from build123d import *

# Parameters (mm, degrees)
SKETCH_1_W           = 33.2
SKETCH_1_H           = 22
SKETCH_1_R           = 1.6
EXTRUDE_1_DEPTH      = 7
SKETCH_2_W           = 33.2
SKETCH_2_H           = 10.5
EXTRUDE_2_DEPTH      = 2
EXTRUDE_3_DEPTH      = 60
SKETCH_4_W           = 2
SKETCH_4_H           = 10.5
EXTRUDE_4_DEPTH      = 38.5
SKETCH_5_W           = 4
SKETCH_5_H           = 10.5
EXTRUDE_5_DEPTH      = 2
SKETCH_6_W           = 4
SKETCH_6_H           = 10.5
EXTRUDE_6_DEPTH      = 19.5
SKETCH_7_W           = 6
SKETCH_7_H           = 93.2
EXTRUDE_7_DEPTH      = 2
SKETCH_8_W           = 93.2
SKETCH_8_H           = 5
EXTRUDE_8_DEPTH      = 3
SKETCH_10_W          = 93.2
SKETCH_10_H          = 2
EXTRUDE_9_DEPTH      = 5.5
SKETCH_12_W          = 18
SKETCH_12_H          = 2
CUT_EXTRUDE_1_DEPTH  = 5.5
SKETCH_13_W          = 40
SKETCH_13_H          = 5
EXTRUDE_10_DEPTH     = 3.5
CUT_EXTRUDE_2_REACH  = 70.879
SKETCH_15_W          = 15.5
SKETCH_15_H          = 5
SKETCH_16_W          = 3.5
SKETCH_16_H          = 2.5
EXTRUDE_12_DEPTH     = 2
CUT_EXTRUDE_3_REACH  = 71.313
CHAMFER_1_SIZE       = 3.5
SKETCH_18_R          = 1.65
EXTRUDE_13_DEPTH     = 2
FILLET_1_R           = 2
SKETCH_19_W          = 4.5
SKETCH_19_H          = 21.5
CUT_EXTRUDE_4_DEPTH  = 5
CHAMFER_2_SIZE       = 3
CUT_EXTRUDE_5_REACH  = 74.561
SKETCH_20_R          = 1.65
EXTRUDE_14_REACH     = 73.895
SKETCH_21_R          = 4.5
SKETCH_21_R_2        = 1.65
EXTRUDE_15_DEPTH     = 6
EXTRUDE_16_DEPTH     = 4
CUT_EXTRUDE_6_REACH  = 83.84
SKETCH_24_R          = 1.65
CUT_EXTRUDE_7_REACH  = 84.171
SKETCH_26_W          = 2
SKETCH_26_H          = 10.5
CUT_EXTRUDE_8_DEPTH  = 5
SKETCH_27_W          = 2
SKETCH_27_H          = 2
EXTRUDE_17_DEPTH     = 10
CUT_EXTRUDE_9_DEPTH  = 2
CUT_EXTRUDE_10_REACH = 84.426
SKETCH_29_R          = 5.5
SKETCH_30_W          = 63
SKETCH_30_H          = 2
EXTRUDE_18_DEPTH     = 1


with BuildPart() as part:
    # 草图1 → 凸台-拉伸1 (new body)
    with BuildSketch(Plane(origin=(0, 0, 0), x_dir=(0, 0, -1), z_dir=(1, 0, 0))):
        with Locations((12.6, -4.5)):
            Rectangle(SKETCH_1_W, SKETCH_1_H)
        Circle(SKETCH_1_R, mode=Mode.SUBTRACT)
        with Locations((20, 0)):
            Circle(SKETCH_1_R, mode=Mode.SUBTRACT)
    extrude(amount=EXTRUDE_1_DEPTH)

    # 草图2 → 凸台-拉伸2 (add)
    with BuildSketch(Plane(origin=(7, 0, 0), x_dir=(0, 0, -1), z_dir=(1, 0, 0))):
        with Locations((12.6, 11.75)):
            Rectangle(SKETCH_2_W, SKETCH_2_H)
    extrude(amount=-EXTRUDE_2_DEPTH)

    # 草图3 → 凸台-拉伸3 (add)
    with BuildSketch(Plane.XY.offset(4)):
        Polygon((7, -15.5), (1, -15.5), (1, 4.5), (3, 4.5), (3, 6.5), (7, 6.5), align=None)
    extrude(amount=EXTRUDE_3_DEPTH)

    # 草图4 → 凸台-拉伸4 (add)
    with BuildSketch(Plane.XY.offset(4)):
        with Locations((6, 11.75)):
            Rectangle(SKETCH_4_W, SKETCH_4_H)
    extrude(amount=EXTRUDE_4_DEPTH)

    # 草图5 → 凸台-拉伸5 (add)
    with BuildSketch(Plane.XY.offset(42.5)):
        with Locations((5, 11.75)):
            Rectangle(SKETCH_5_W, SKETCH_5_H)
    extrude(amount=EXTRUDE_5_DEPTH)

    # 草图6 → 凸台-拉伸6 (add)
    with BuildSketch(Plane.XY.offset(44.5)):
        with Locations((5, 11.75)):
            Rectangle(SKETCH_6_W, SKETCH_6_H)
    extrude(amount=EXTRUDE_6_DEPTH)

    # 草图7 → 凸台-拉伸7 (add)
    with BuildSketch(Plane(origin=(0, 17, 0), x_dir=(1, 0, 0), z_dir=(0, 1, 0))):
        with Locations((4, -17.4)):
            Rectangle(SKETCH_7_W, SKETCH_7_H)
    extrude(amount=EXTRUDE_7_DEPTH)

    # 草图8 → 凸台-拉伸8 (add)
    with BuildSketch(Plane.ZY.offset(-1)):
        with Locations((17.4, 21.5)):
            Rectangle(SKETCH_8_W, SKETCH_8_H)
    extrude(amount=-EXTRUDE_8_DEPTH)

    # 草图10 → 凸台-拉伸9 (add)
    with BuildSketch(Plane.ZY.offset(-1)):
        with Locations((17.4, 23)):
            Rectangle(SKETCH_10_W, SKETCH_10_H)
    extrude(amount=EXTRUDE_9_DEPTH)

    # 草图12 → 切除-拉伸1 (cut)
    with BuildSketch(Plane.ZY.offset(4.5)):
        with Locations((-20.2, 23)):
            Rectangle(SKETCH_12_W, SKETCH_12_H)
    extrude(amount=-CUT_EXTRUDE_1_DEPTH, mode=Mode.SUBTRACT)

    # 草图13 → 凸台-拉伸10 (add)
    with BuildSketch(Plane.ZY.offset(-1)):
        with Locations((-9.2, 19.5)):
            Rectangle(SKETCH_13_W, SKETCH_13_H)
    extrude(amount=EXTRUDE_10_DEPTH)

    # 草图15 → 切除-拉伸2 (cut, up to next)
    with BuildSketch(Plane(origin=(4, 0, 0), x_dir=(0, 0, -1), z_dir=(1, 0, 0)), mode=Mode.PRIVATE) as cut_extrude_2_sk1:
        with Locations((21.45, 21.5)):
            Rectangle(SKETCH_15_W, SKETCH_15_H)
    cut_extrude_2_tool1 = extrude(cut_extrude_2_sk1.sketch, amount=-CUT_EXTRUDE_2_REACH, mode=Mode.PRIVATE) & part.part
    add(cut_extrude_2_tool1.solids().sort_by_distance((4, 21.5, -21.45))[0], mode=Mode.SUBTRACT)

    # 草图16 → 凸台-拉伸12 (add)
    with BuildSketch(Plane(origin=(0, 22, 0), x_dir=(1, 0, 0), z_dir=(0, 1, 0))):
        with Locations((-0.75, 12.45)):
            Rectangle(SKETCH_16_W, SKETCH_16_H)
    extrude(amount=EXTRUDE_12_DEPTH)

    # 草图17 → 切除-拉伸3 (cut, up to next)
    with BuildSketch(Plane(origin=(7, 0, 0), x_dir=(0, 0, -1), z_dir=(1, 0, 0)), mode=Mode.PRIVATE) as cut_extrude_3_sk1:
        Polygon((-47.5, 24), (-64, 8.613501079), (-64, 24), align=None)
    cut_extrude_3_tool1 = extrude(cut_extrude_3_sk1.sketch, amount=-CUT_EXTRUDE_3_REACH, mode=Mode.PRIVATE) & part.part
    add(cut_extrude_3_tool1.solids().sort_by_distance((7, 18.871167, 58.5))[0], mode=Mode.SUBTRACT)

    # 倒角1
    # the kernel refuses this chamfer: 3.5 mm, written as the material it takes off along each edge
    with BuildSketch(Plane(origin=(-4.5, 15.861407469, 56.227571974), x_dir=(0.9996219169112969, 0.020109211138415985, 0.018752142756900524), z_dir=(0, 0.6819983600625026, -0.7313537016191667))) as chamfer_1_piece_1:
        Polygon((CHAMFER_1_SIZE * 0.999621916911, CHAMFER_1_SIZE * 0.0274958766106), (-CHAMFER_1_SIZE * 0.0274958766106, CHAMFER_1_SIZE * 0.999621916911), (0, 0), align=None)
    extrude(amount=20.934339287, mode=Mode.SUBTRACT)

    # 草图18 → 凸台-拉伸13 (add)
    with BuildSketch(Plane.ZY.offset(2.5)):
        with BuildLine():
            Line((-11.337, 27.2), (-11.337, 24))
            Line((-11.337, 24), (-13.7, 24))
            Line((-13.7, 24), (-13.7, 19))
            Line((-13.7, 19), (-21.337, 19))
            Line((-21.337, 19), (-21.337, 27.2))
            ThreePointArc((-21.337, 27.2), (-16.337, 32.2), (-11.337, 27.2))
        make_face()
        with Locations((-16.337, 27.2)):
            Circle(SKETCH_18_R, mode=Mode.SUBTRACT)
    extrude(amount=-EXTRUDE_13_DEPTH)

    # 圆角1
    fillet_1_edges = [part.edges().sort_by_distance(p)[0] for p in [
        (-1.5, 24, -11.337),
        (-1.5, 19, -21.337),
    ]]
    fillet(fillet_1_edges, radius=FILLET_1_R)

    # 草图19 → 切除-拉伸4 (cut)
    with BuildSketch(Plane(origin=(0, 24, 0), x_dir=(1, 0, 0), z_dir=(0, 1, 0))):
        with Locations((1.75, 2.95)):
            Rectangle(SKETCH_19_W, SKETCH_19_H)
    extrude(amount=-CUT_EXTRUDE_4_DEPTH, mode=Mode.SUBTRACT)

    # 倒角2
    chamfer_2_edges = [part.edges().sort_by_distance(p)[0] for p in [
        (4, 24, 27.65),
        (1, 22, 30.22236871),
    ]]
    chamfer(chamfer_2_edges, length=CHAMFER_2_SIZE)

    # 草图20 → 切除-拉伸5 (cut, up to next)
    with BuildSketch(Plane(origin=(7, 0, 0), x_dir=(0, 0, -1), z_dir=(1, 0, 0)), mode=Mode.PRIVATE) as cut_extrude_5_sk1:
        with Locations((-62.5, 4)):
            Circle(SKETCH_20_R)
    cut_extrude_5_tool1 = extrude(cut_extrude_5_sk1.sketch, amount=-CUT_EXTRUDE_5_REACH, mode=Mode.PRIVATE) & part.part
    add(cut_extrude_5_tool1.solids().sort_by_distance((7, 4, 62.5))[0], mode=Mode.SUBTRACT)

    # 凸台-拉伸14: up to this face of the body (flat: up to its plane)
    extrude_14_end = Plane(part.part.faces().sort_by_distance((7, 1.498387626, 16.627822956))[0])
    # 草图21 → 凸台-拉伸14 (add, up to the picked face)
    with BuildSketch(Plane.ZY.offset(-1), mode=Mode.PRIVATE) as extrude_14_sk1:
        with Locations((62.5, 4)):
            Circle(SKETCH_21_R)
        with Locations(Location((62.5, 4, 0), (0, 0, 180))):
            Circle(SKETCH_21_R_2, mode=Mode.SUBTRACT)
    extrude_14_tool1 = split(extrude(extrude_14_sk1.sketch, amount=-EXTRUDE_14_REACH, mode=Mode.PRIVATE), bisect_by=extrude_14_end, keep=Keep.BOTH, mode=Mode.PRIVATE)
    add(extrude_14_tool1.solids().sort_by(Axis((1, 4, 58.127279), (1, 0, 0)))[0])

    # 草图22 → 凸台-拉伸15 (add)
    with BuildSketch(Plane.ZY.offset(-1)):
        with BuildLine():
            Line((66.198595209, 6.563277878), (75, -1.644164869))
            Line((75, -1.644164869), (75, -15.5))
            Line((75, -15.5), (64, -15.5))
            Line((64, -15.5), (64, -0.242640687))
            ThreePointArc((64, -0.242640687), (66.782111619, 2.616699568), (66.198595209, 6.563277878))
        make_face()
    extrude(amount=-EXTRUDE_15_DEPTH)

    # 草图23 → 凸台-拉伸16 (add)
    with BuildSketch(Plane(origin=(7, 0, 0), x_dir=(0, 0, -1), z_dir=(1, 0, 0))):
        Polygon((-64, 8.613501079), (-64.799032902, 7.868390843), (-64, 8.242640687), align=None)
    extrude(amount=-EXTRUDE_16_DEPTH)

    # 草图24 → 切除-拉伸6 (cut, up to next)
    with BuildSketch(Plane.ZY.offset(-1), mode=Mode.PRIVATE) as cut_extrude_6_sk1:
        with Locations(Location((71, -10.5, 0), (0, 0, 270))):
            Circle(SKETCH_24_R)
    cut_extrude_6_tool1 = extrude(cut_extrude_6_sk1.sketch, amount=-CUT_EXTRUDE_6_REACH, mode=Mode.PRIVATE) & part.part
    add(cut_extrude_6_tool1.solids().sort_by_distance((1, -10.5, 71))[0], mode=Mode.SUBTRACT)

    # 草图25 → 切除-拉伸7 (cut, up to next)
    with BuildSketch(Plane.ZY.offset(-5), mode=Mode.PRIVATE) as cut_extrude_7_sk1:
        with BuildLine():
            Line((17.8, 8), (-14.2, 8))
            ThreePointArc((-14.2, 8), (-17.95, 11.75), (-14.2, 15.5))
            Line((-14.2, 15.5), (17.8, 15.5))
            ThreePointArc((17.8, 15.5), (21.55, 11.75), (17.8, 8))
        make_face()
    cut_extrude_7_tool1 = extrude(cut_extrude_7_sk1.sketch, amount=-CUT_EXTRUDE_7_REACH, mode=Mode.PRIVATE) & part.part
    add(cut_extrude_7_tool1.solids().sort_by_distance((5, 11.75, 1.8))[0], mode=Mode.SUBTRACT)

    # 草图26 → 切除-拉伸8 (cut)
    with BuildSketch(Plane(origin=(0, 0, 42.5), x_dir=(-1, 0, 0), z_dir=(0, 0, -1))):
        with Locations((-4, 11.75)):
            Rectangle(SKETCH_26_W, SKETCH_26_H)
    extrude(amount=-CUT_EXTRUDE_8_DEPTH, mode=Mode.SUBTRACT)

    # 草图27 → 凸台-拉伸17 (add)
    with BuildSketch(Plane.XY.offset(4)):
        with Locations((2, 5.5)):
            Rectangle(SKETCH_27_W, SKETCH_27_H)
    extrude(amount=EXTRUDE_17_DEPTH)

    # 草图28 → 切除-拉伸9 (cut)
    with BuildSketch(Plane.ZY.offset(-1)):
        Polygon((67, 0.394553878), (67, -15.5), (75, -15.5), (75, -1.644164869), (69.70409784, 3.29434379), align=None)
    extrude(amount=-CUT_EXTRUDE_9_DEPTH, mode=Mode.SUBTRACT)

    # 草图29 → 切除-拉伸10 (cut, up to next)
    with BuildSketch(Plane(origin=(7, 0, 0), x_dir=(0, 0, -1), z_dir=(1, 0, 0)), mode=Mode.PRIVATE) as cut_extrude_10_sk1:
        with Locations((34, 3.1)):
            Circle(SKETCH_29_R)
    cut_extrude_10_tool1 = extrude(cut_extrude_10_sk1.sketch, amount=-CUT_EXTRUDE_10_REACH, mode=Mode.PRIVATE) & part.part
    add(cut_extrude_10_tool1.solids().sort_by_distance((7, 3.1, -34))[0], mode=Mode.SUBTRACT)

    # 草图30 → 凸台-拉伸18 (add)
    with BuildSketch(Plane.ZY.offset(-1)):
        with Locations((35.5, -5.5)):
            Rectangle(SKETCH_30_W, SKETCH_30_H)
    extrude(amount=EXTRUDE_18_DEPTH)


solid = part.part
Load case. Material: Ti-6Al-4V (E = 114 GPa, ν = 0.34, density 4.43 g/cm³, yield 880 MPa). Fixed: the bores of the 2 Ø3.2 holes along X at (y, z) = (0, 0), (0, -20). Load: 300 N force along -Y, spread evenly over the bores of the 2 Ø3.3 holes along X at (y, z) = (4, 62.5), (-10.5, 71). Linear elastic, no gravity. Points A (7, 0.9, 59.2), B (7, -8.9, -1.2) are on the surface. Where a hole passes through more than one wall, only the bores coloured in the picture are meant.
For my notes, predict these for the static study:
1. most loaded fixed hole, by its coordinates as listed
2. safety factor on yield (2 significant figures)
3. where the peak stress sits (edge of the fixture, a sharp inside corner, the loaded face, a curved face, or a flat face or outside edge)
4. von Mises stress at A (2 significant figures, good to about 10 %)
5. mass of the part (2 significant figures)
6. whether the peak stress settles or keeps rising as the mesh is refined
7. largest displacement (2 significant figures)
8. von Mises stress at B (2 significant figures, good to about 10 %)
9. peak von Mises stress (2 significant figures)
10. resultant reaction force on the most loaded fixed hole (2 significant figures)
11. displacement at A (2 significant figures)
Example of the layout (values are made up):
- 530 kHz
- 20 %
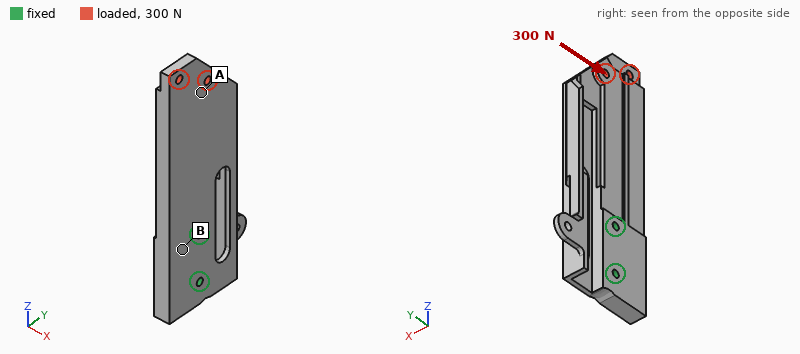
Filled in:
- (0, 0)
- 11
- a curved face
- 4.7 MPa
- 81 g
- settles
- 57 µm
- 16 MPa
- 82 MPa
- 1.1 kN
- 42 µm
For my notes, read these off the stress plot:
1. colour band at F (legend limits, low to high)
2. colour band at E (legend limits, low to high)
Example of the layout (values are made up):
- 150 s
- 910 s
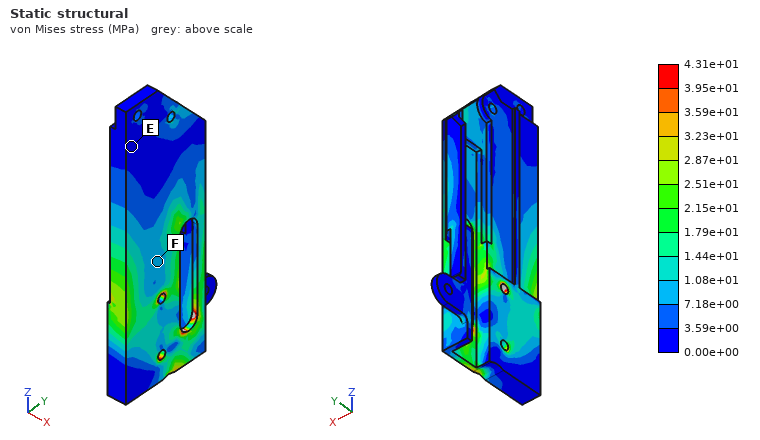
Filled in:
- 7.18e+00 to 1.08e+01 MPa
- 0.00e+00 to 3.59e+00 MPa
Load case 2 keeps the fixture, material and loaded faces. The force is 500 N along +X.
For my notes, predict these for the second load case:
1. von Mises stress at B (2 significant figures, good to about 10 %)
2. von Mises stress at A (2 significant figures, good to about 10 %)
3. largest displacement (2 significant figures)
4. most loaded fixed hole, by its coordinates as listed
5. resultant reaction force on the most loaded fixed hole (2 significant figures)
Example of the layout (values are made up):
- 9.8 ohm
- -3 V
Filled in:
- 81 MPa
- 45 MPa
- 0.90 mm
- (0, 0)
- 1.2 kN
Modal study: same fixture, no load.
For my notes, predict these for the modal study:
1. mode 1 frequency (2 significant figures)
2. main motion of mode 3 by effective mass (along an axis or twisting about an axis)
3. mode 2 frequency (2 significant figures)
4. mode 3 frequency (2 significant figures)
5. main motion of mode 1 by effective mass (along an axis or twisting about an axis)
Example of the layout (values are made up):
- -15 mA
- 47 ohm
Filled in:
- 1000 Hz
- along Y
- 1900 Hz
- 2800 Hz
- along X
